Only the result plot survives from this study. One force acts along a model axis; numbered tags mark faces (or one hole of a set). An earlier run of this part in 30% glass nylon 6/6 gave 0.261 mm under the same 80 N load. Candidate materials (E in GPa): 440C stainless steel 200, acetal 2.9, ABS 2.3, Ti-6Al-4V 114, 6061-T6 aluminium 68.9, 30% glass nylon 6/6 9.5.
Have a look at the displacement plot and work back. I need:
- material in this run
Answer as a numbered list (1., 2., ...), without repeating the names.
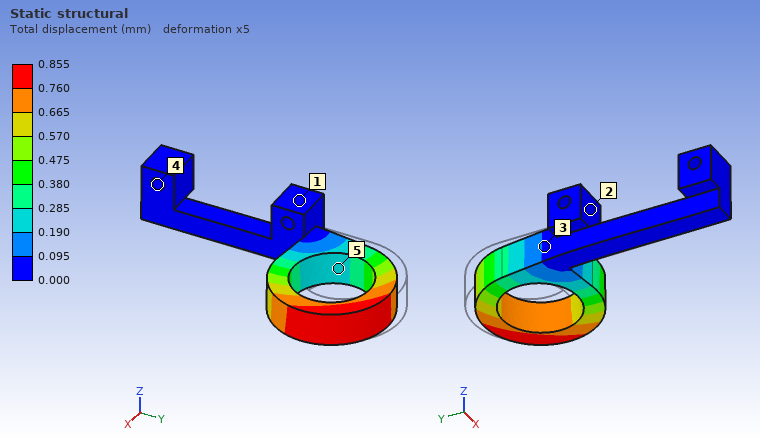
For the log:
1. acetal
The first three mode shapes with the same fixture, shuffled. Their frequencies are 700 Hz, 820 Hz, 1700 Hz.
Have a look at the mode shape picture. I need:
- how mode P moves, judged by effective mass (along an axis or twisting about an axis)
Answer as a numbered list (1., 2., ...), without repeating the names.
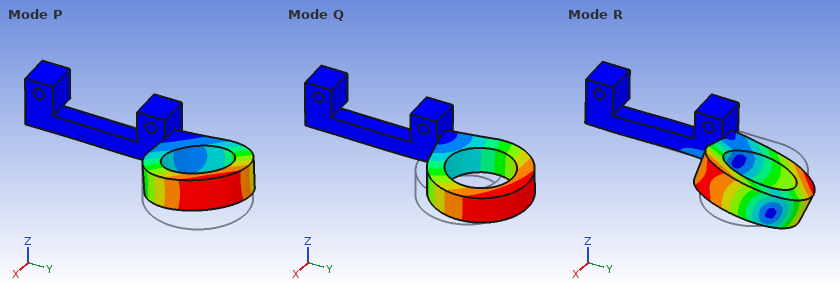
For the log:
1. along Z
